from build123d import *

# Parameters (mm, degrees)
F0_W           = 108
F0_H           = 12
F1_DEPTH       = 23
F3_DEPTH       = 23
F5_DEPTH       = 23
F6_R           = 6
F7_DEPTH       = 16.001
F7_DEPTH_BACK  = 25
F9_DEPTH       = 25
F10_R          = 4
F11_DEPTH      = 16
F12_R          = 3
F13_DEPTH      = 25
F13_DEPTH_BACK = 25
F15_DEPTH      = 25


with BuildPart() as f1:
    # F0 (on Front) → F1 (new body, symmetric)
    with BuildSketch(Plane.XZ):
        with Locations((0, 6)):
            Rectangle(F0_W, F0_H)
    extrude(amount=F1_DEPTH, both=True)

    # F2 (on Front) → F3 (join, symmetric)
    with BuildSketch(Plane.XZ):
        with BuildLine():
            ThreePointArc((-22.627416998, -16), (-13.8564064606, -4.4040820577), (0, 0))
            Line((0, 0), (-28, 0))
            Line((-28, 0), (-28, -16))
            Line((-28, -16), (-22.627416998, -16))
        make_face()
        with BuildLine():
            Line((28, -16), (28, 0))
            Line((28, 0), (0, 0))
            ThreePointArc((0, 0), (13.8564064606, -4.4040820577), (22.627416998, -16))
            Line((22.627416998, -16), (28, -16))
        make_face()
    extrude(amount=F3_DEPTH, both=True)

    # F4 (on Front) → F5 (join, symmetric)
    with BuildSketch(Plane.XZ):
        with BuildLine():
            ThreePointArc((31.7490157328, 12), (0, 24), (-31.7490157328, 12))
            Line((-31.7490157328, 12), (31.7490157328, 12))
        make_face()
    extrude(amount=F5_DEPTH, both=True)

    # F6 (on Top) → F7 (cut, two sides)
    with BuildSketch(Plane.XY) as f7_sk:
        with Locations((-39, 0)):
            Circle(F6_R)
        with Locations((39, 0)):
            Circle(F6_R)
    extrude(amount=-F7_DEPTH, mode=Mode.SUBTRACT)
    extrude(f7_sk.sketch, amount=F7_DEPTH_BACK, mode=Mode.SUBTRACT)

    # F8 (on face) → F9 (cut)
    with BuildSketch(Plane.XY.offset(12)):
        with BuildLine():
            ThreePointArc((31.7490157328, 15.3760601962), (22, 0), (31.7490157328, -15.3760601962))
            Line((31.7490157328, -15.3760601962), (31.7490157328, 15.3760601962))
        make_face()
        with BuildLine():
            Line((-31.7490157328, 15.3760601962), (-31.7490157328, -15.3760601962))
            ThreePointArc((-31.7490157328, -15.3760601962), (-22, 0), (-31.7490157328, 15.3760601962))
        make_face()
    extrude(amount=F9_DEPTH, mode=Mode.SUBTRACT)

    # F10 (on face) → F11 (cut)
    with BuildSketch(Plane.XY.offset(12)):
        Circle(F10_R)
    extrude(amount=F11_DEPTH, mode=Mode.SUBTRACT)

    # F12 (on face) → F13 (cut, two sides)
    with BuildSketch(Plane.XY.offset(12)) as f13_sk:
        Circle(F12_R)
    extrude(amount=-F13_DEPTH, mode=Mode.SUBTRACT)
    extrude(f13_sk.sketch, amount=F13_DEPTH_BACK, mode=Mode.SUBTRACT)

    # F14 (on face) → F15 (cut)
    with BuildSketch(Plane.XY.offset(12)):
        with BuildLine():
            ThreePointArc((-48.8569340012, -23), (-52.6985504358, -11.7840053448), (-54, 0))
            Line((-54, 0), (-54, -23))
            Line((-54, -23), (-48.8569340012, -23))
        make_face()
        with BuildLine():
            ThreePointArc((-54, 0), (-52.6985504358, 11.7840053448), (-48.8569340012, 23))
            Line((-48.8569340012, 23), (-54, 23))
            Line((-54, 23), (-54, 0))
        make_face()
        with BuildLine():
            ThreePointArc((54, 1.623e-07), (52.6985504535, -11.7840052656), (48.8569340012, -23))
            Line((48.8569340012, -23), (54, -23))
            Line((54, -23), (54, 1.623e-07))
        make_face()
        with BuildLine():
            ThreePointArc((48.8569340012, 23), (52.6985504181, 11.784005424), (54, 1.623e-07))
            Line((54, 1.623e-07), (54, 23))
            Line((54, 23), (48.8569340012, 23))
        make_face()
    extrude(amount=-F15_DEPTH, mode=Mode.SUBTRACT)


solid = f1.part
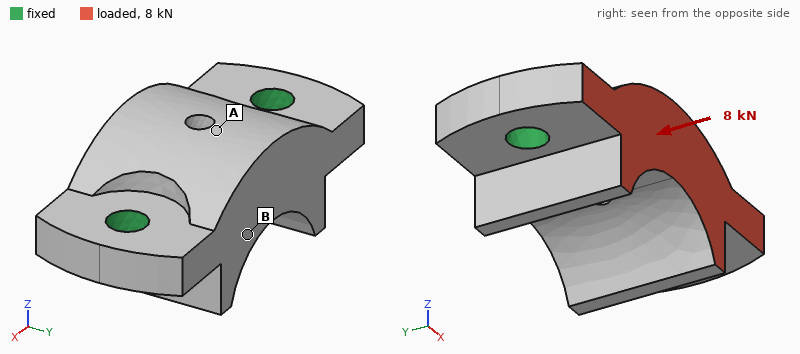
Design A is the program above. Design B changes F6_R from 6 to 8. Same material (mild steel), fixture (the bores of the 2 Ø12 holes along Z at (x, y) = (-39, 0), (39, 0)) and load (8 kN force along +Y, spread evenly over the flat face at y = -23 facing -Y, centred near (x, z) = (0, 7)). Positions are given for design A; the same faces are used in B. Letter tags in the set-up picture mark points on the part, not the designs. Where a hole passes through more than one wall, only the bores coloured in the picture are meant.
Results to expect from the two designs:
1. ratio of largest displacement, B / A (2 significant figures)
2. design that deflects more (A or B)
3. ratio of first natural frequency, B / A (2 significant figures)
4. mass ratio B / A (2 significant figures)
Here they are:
0.84
A
1.2
0.98
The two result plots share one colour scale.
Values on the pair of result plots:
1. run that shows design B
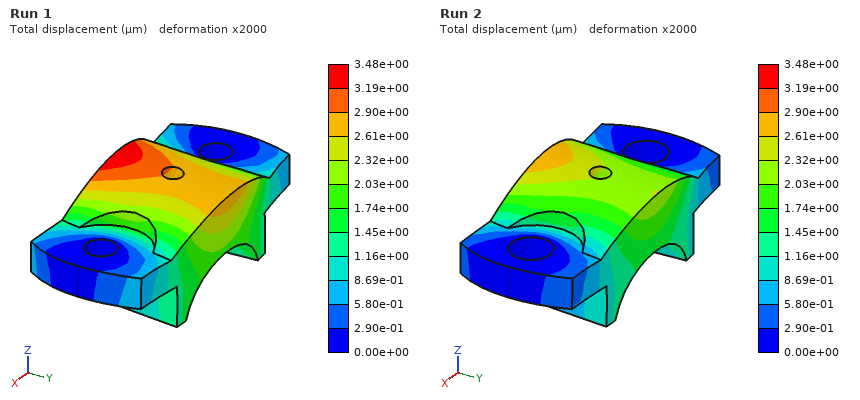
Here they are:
Run 2
